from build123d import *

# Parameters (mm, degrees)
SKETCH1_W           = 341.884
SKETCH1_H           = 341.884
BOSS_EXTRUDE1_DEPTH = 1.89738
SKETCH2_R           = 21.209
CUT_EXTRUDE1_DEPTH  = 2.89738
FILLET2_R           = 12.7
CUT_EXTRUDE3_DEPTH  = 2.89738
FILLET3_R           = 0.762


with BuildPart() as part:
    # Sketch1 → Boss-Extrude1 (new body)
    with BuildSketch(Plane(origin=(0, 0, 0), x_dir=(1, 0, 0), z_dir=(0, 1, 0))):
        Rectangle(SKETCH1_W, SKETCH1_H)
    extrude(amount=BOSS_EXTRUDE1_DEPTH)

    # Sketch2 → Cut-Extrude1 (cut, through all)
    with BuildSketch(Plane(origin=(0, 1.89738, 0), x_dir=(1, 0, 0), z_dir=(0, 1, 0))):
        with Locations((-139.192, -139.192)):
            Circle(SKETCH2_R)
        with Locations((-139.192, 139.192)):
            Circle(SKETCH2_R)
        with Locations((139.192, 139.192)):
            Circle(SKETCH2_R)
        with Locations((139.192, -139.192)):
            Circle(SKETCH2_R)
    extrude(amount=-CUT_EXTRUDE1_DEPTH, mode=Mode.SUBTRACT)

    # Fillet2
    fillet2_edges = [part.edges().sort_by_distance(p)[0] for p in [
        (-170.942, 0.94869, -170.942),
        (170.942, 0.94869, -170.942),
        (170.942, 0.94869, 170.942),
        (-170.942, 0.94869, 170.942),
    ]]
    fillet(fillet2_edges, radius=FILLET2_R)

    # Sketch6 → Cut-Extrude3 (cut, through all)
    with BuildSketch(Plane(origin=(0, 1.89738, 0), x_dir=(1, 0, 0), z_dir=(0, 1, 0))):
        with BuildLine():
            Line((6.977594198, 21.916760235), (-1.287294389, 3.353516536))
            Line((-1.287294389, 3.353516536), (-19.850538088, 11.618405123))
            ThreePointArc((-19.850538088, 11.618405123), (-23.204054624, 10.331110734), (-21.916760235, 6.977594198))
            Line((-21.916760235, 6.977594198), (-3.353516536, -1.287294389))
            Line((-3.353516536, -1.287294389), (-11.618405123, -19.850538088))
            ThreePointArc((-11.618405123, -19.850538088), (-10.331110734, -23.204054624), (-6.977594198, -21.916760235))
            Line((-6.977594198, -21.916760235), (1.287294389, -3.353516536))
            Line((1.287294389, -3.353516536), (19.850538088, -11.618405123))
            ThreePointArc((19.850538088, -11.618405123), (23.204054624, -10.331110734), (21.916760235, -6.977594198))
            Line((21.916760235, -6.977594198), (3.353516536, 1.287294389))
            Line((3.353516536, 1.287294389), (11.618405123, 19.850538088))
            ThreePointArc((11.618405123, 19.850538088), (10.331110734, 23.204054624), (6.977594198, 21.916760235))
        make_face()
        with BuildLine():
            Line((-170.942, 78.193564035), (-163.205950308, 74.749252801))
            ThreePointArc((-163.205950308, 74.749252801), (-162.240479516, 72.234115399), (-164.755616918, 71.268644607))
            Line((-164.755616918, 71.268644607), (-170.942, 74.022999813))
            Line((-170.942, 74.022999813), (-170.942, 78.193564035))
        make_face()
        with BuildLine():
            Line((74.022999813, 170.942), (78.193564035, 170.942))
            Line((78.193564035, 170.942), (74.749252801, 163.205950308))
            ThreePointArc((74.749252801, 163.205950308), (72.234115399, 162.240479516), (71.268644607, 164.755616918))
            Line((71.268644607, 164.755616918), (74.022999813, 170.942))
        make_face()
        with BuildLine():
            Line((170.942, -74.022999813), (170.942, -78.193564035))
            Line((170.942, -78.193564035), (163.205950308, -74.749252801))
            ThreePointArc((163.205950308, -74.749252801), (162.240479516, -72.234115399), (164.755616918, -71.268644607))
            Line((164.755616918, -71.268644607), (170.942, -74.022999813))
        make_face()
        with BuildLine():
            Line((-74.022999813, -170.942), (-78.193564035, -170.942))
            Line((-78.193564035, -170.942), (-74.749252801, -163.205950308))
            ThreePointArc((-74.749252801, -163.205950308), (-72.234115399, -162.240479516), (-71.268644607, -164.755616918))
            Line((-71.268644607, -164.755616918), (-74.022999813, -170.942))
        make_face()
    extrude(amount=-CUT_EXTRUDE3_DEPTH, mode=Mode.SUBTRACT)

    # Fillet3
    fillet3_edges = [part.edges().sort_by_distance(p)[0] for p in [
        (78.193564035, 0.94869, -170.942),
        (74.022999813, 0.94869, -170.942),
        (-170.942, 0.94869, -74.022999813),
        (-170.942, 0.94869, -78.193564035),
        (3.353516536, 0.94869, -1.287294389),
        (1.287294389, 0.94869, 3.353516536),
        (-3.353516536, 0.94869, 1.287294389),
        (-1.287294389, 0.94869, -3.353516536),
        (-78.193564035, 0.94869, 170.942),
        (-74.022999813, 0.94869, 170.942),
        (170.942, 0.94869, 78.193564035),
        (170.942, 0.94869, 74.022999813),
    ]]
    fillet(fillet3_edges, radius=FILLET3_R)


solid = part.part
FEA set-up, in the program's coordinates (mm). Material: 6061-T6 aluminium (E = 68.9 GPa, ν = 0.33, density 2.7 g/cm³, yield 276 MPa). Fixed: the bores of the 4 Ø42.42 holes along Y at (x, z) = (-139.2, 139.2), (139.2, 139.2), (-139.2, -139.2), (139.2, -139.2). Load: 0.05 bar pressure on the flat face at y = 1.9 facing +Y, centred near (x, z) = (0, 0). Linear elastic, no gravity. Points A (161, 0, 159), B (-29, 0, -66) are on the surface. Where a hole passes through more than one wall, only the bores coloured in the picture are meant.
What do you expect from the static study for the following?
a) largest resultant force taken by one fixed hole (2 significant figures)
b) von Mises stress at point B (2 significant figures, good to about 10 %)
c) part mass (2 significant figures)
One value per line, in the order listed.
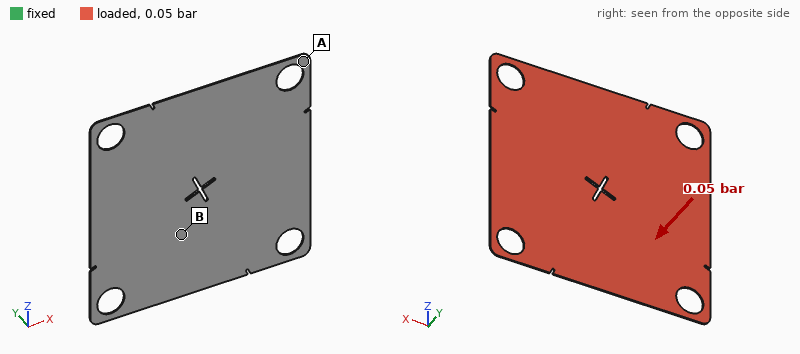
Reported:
140 N
21 MPa
570 g
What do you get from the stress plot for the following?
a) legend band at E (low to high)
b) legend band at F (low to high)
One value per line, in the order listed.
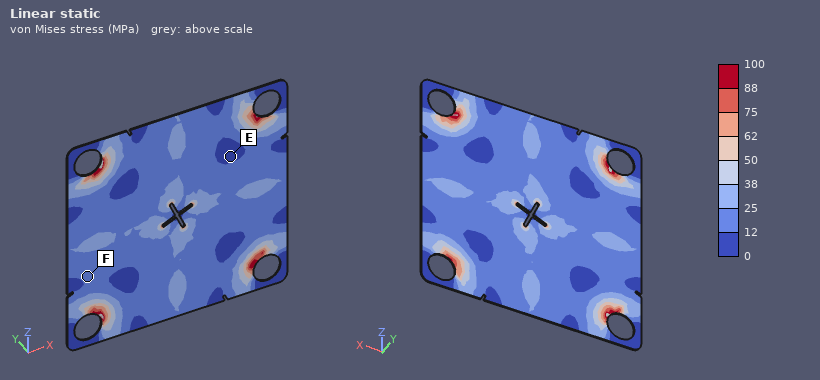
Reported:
0 to 12 MPa
12 to 25 MPa
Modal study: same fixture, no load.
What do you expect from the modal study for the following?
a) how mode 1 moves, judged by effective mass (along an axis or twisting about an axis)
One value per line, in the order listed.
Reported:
along Y
